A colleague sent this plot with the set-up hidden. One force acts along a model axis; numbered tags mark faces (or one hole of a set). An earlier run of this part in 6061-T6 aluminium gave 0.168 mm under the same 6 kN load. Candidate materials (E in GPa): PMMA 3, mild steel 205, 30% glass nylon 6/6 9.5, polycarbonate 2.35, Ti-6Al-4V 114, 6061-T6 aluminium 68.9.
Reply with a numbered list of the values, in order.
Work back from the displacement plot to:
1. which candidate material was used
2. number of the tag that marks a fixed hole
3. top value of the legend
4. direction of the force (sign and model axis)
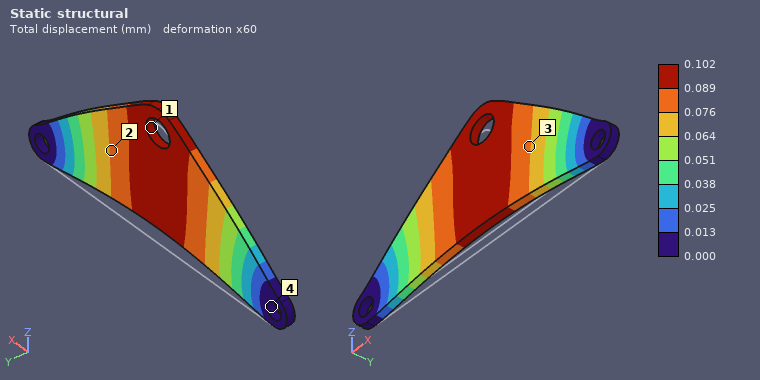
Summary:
1. Ti-6Al-4V
2. 4
3. 0.102 mm
4. +Z
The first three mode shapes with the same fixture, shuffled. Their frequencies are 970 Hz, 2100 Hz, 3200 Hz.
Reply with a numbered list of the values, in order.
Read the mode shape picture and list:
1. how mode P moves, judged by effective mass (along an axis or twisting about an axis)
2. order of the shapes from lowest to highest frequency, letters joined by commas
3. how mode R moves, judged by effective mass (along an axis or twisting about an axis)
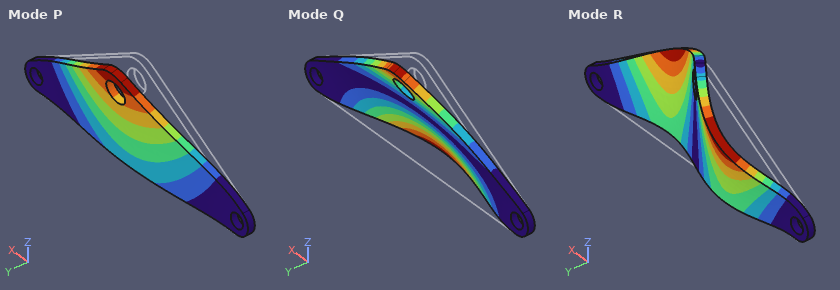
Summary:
1. along Y
2. P, Q, R
3. twisting about Z
